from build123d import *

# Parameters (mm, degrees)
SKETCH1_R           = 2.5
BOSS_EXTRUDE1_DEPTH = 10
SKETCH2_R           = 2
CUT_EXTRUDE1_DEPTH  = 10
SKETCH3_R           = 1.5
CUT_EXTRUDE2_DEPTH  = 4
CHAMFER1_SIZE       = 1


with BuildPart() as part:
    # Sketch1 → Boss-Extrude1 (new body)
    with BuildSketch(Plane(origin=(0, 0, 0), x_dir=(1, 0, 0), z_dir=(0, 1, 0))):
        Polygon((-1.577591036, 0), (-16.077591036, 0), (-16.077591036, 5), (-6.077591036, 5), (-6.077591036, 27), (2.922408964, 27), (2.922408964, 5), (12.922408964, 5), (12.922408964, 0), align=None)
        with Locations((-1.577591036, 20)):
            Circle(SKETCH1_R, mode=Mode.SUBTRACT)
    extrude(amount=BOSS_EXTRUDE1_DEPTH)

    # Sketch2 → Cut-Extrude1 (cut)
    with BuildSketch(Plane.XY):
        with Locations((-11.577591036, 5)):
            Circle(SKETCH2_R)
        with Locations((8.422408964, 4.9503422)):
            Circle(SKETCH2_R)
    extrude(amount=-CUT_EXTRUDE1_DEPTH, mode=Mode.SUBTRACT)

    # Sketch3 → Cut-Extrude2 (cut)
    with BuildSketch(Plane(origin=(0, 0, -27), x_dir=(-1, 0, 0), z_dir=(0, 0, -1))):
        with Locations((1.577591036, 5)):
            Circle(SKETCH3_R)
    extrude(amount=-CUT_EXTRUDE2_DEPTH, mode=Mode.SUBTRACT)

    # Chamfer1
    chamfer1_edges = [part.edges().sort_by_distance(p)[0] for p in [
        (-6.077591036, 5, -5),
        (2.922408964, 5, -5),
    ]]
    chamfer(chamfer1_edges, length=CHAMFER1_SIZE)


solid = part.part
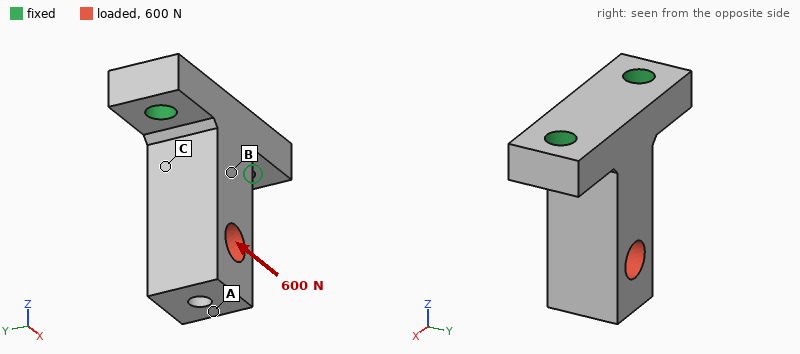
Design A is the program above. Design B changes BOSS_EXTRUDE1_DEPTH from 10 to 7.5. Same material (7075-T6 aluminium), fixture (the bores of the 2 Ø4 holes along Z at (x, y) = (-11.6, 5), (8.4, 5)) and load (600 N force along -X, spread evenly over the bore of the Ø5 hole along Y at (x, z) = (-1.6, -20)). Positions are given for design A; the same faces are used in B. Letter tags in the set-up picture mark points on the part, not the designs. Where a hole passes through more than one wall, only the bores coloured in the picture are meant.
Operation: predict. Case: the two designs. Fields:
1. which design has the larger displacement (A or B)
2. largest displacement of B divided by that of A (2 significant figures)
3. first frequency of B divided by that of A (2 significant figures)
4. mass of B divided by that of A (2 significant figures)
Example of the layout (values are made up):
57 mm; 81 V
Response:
B; 1.3; 0.88; 0.74
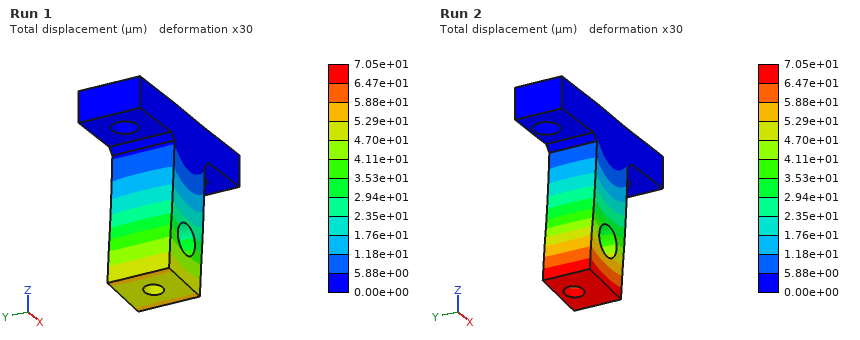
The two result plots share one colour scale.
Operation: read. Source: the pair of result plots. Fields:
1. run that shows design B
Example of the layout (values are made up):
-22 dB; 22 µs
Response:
Run 2
